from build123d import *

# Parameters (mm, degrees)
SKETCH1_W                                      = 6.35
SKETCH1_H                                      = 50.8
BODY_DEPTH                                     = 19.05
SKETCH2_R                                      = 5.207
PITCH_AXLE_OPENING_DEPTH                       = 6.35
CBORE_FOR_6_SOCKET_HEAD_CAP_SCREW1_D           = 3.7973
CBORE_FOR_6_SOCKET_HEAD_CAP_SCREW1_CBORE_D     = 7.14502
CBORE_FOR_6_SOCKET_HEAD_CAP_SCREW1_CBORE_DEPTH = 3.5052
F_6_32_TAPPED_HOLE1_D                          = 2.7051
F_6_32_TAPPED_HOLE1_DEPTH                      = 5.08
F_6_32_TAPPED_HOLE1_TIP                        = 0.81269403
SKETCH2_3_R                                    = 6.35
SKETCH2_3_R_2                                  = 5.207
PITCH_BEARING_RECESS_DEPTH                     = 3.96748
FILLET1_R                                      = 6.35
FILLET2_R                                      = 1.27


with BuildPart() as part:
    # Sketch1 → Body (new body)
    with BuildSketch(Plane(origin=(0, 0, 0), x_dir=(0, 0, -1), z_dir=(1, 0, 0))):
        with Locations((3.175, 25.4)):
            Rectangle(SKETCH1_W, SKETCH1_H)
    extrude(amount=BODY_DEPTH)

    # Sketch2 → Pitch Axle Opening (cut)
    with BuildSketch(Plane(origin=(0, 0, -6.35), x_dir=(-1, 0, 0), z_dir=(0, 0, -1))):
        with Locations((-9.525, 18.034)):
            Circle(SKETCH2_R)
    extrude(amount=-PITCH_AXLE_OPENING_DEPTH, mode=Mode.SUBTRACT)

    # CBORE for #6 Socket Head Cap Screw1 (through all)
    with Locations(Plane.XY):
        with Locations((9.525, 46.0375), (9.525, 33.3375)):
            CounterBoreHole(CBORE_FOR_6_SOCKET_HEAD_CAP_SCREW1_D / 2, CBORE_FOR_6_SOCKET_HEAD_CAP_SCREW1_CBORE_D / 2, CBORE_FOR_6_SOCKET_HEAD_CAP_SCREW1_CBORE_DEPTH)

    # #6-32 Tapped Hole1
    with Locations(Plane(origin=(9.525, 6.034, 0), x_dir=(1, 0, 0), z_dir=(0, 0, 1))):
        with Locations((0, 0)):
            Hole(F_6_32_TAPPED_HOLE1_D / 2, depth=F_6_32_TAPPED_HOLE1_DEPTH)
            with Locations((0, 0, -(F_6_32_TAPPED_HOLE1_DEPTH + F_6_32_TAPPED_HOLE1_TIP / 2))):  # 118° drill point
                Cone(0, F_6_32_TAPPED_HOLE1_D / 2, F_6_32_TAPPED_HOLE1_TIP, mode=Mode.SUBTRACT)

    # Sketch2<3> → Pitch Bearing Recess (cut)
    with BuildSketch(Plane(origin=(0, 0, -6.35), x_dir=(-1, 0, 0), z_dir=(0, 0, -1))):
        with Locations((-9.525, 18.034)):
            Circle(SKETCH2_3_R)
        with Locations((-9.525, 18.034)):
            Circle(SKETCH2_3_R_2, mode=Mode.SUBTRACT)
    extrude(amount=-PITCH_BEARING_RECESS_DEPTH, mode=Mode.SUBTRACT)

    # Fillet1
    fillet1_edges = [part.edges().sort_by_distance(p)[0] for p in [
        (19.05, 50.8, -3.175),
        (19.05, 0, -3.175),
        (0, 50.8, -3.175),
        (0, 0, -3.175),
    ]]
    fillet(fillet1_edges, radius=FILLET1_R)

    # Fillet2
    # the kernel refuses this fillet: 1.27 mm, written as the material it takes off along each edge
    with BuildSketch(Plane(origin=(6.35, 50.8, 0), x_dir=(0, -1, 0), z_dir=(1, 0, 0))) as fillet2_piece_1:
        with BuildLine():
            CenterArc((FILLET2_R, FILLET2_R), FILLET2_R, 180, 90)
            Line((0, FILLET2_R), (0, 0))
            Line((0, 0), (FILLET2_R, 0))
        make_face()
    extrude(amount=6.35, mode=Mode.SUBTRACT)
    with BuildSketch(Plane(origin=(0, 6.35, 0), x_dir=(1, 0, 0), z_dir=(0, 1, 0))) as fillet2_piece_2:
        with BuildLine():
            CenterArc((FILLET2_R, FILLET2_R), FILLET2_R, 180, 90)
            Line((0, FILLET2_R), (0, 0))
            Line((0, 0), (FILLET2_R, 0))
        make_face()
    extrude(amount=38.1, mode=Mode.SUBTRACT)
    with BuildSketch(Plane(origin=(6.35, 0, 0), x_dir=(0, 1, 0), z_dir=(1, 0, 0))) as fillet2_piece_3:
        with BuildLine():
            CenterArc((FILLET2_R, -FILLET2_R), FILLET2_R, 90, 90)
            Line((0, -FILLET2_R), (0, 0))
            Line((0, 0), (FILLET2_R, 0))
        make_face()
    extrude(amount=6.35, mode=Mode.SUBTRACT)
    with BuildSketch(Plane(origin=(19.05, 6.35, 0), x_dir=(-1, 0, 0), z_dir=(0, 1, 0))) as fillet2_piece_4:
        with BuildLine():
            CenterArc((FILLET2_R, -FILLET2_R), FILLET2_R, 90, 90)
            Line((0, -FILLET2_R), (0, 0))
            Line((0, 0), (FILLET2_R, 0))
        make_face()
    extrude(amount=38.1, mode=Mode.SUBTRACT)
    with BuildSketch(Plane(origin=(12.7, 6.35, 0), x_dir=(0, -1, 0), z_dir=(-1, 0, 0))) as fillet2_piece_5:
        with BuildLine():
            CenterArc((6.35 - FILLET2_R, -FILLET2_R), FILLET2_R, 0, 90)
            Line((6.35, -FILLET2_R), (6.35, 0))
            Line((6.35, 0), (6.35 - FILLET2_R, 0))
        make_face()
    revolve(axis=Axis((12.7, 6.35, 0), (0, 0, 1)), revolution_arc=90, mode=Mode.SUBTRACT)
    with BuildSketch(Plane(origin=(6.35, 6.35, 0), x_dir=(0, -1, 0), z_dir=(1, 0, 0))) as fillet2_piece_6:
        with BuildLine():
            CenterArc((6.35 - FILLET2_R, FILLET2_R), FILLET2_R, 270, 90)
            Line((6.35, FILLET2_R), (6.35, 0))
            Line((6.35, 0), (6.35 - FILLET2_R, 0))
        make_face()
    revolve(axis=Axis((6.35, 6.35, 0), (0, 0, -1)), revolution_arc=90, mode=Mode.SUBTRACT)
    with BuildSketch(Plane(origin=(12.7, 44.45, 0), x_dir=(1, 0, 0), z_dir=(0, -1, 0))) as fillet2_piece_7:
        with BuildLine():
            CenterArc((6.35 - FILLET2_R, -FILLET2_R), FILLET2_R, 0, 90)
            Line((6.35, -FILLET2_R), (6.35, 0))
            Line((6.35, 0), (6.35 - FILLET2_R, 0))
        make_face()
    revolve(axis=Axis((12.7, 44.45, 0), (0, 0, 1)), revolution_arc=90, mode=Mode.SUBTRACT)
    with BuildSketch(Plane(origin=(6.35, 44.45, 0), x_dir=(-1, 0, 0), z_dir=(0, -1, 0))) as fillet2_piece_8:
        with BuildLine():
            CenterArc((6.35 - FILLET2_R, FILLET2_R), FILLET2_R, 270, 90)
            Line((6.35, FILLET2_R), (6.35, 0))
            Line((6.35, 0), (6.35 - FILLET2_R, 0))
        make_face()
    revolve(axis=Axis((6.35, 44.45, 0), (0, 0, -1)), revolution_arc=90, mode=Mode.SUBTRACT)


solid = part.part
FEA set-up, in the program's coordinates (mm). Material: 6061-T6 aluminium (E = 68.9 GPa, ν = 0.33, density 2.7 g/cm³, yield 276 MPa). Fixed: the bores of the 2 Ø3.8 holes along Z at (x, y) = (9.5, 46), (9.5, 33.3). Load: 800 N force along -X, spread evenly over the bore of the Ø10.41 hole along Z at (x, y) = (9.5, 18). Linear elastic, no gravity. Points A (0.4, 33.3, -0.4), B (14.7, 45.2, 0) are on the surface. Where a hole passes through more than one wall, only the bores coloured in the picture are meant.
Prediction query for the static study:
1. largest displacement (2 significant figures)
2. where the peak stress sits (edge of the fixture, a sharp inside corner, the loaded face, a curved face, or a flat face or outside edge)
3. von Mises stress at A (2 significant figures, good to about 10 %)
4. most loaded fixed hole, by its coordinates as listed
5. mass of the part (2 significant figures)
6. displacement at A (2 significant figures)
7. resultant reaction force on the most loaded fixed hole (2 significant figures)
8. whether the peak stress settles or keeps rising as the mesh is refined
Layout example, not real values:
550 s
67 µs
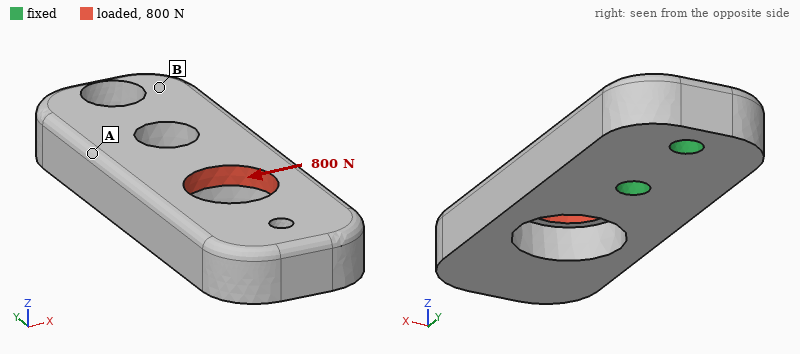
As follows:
60 µm
edge of the fixture
27 MPa
(9.5, 33.3)
13 g
13 µm
1.5 kN
keeps rising
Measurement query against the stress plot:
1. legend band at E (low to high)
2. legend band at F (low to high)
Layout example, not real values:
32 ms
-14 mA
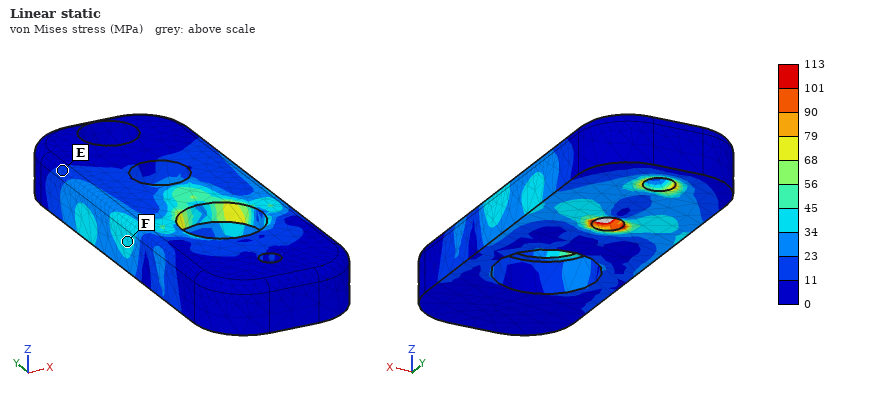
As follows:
11 to 23 MPa
34 to 45 MPa
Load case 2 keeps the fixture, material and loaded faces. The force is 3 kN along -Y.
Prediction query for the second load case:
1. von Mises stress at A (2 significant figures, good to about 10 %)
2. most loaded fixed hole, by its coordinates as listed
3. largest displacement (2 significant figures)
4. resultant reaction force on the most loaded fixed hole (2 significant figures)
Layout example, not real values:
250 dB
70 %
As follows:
72 MPa
(9.5, 33.3)
0.18 mm
1.8 kN
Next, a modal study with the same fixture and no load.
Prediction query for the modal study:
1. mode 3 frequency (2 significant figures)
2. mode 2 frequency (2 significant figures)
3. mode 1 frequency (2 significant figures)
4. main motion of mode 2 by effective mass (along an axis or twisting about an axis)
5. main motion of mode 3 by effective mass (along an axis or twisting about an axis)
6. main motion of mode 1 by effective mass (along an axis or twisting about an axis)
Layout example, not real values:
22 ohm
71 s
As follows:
9400 Hz
7200 Hz
3600 Hz
along X
twisting about Y
along Z
